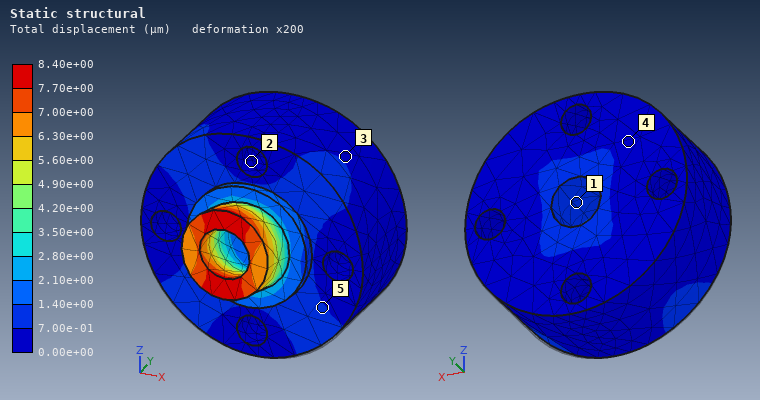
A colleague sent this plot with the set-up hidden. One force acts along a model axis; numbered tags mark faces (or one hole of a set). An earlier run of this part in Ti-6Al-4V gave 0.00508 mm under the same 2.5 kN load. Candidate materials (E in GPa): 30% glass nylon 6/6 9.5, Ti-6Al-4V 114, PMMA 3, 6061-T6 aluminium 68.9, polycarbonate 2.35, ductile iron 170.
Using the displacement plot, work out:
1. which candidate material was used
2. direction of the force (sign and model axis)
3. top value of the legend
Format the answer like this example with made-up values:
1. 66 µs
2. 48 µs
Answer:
1. 6061-T6 aluminium
2. +Z
3. 8.40e+00 µm
